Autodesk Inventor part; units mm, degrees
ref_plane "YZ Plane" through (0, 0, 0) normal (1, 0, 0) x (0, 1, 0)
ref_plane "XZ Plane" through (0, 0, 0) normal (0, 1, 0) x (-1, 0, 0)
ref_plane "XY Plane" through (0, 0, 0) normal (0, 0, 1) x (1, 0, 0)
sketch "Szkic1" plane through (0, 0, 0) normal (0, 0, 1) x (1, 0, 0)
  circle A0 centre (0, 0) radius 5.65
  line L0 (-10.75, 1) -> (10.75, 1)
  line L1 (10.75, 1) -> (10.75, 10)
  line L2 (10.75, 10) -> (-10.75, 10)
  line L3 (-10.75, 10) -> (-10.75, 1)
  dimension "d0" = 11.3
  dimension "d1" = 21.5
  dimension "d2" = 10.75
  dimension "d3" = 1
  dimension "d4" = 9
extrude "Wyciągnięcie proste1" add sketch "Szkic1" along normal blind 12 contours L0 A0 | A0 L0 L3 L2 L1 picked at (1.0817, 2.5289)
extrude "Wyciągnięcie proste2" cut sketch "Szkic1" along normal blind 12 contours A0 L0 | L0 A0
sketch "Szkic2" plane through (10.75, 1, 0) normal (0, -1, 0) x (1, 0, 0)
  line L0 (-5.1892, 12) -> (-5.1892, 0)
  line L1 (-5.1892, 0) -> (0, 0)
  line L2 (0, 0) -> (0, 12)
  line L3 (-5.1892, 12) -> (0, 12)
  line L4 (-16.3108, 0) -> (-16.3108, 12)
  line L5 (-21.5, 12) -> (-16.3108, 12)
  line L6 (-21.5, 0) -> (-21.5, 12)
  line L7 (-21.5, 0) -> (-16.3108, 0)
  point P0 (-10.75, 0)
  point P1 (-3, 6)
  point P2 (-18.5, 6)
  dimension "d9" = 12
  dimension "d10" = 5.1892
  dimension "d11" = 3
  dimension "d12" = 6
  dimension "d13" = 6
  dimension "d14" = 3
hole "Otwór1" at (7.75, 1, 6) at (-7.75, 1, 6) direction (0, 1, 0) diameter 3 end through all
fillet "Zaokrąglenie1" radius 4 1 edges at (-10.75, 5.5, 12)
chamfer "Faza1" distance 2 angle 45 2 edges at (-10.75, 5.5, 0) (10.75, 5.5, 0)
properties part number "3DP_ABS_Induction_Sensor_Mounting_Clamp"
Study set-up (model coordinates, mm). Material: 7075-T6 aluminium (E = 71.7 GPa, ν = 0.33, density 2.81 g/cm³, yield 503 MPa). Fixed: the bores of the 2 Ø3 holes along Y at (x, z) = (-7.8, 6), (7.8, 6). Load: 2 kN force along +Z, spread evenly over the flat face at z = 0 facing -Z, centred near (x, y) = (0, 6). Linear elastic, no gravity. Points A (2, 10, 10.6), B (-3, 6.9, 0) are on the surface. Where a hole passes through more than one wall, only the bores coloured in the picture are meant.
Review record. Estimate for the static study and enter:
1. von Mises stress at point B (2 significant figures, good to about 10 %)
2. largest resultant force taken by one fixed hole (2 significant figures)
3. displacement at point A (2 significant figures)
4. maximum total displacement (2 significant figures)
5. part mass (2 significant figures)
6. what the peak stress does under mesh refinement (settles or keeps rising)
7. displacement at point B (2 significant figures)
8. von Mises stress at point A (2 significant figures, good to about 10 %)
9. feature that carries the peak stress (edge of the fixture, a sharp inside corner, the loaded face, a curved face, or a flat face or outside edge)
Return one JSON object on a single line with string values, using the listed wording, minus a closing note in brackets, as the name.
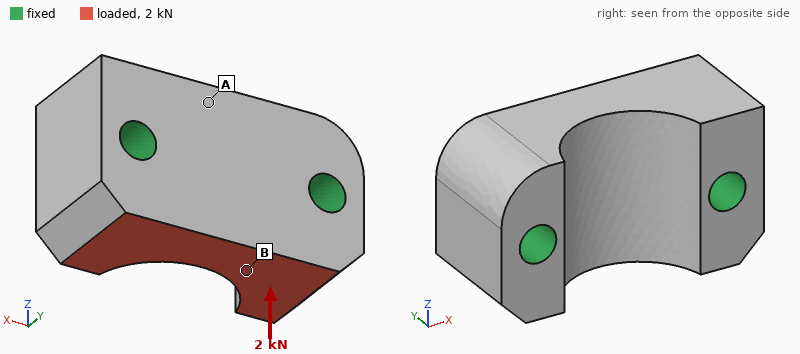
{"von Mises stress at point B": "17 MPa", "largest resultant force taken by one fixed hole": "1.0 kN", "displacement at point A": "1.8 µm", "maximum total displacement": "3.5 µm", "part mass": "4.7 g", "what the peak stress does under mesh refinement": "keeps rising", "displacement at point B": "2.5 µm", "von Mises stress at point A": "8.7 MPa", "feature that carries the peak stress": "edge of the fixture"}
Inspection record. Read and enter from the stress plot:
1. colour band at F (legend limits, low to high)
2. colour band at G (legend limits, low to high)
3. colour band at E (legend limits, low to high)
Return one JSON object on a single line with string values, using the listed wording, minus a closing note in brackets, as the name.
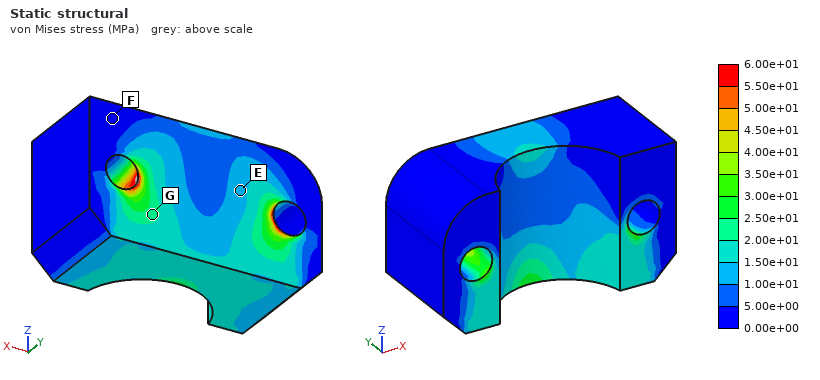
{"colour band at F": "0.00e+00 to 5.00e+00 MPa", "colour band at G": "2.00e+01 to 2.50e+01 MPa", "colour band at E": "1.00e+01 to 1.50e+01 MPa"}
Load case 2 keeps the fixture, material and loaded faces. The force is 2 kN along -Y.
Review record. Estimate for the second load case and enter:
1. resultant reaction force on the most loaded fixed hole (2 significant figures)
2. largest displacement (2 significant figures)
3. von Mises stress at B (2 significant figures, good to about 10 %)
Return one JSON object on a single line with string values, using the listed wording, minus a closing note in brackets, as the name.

{"resultant reaction force on the most loaded fixed hole": "1.0 kN", "largest displacement": "12 µm", "von Mises stress at B": "53 MPa"}
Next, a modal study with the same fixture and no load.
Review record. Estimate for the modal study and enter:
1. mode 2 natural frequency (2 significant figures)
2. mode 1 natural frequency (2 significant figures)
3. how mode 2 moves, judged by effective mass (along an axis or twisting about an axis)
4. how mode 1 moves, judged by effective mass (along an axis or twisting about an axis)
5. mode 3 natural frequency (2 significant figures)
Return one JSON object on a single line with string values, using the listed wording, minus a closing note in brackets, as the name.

{"mode 2 natural frequency": "85 kHz", "mode 1 natural frequency": "79 kHz", "how mode 2 moves, judged by effective mass": "along Y", "how mode 1 moves, judged by effective mass": "along Z", "mode 3 natural frequency": "98 kHz"}
